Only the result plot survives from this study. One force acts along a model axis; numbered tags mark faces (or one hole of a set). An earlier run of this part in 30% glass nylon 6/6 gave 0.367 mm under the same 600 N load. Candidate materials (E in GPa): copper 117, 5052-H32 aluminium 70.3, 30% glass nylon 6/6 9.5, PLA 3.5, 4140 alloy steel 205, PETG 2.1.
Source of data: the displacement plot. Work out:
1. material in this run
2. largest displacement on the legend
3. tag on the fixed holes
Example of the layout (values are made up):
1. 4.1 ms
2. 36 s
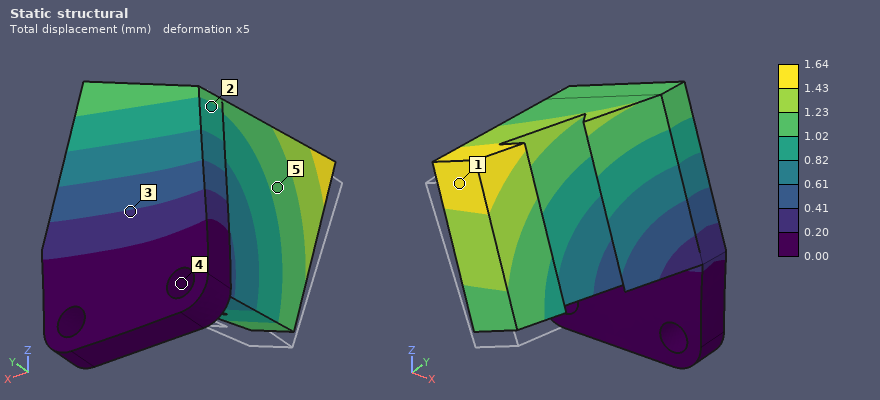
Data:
1. PETG
2. 1.64 mm
3. 4
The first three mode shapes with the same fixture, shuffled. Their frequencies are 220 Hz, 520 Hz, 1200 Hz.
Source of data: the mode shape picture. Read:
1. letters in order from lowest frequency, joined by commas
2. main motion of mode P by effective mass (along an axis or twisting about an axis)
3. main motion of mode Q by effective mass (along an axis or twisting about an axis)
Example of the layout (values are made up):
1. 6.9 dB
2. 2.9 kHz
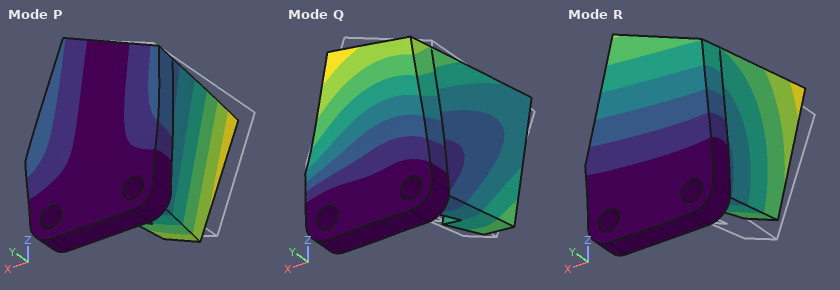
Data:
1. R, P, Q
2. along X
3. along X
